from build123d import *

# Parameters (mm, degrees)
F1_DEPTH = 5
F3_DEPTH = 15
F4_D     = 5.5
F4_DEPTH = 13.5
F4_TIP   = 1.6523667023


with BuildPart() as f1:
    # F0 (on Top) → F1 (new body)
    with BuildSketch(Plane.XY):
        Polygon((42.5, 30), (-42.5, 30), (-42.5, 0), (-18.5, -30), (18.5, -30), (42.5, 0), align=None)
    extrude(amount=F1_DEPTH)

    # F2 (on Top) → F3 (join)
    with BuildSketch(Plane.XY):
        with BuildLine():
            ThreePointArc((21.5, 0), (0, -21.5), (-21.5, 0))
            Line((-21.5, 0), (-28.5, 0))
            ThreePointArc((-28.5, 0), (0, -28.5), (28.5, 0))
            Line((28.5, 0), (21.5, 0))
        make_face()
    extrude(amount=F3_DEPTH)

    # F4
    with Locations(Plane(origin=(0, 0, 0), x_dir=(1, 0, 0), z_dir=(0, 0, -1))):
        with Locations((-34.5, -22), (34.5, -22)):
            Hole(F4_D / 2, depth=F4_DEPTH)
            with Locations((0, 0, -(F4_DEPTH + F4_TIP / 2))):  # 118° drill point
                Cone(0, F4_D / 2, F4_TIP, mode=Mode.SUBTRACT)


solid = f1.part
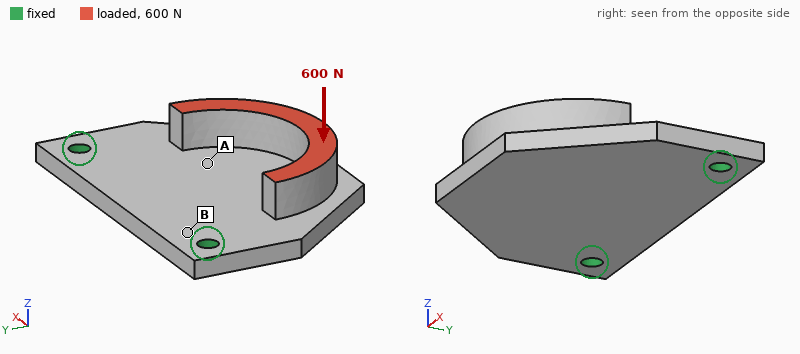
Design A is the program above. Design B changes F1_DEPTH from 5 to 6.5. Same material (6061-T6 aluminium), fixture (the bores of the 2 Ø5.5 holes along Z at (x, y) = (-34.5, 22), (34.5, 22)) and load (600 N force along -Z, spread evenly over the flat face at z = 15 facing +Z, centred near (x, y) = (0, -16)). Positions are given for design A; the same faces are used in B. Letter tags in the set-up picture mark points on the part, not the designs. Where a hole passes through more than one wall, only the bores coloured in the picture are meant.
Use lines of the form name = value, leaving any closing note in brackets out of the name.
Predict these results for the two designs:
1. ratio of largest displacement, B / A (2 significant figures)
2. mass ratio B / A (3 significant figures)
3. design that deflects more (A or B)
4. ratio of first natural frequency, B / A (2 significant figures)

ratio of largest displacement, B / A = 0.50
mass ratio B / A = 1.21
design that deflects more = A
ratio of first natural frequency, B / A = 1.3
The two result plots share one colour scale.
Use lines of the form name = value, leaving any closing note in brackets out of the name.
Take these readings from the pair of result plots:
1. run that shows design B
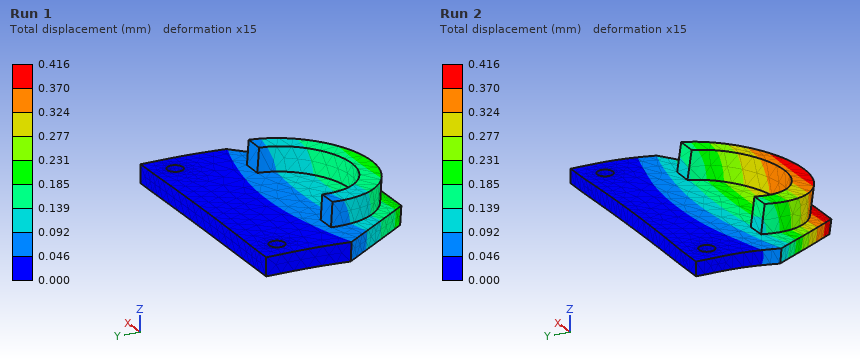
run that shows design B = Run 1
